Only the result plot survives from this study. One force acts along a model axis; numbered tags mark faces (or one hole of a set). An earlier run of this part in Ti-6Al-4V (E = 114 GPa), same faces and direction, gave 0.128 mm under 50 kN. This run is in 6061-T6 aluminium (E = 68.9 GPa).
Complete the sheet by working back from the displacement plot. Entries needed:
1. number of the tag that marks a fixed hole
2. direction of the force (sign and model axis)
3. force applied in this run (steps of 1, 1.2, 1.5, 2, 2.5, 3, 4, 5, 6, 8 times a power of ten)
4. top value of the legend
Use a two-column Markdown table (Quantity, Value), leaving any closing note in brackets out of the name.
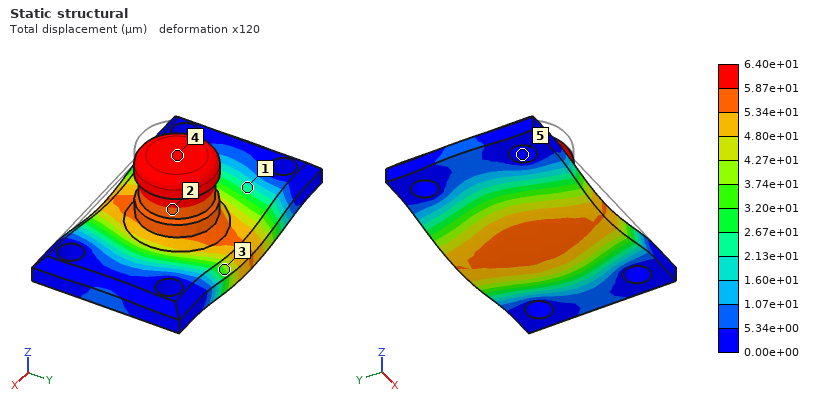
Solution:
| Quantity | Value |
|---|---|
| number of the tag that marks a fixed hole | 5 |
| direction of the force | -Z |
| force applied in this run | 15 kN |
| top value of the legend | 6.40e+01 µm |
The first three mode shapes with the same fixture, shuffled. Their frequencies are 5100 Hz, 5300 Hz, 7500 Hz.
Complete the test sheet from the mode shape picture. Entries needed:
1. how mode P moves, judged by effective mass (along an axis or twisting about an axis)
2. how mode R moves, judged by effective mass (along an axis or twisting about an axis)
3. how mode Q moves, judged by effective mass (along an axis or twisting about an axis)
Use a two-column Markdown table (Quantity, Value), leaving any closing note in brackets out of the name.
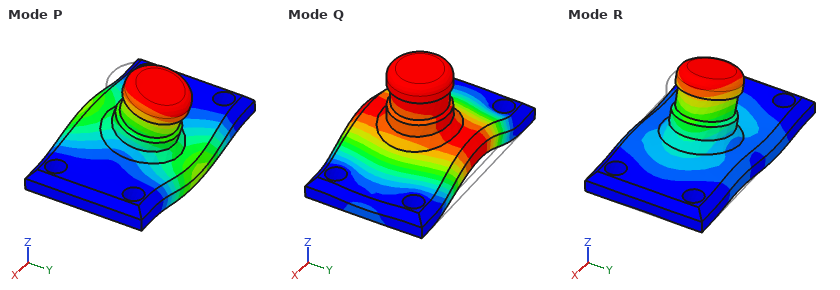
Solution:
| Quantity | Value |
|---|---|
| how mode P moves, judged by effective mass | along Y |
| how mode R moves, judged by effective mass | along X |
| how mode Q moves, judged by effective mass | along Z |
